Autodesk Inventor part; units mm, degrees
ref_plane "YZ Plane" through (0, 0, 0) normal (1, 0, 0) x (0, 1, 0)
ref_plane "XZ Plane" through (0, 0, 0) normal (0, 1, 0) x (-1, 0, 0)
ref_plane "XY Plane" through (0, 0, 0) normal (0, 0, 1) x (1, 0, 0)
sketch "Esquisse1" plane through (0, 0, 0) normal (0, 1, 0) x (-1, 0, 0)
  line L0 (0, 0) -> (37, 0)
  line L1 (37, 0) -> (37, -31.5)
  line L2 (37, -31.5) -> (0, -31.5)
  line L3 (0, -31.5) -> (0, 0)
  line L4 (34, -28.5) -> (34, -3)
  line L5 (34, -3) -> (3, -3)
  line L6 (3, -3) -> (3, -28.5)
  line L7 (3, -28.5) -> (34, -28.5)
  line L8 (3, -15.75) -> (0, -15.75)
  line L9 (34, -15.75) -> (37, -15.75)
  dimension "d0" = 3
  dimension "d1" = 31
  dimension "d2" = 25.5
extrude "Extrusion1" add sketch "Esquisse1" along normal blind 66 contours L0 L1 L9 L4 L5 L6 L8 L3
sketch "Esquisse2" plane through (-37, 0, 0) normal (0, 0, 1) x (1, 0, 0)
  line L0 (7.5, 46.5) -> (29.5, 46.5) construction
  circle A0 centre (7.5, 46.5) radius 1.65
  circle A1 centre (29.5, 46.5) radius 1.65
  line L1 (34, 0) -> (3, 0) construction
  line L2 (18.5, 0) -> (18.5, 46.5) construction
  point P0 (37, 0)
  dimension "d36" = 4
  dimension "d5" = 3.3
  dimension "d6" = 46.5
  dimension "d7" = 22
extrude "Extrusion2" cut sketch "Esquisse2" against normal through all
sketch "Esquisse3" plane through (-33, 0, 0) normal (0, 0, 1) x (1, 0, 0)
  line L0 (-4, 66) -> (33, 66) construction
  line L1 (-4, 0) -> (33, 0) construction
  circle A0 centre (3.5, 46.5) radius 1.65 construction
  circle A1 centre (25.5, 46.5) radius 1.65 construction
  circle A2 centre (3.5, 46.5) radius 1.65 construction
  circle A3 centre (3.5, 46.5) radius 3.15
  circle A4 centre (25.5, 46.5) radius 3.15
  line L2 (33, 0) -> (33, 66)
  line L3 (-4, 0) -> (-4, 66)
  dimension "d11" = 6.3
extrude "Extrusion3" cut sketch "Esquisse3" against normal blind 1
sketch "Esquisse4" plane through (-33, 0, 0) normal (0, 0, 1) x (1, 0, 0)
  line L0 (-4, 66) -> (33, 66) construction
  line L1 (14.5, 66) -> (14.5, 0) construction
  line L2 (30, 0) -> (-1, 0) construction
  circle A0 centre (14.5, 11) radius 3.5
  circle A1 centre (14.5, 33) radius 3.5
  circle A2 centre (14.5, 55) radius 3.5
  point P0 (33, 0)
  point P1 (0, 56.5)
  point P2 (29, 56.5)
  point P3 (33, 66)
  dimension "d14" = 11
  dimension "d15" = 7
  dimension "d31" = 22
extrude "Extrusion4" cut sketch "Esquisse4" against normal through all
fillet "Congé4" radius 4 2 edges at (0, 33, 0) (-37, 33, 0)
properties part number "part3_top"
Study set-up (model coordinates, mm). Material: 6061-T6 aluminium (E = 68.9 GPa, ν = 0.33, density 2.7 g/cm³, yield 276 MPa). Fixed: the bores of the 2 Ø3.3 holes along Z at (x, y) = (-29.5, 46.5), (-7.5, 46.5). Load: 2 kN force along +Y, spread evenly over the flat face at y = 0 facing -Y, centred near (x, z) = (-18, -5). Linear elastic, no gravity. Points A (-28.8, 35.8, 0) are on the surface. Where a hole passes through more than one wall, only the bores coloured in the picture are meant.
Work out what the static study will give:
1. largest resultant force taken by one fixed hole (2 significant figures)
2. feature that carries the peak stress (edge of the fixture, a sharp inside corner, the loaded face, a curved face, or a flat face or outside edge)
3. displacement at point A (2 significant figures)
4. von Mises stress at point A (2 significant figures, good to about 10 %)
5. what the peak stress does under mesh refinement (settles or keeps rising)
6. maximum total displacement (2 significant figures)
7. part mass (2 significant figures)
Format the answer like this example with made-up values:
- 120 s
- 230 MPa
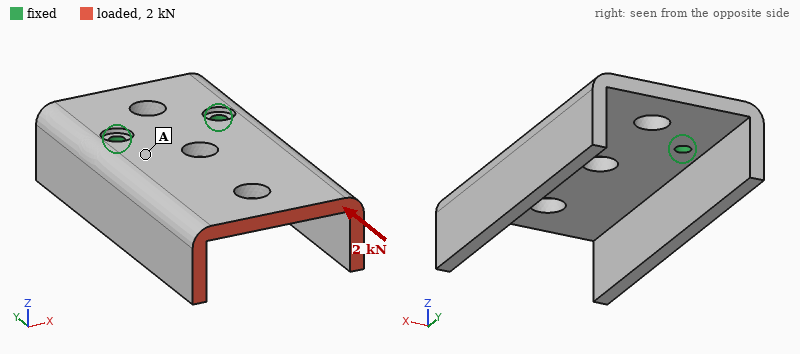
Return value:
- 1.0 kN
- edge of the fixture
- 0.045 mm
- 19 MPa
- keeps rising
- 0.25 mm
- 31 g
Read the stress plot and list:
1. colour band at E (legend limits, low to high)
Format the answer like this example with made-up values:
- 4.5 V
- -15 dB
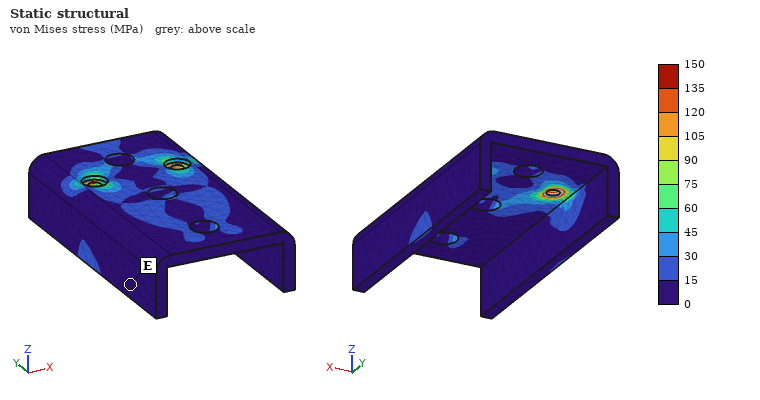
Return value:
- 0 to 15 MPa
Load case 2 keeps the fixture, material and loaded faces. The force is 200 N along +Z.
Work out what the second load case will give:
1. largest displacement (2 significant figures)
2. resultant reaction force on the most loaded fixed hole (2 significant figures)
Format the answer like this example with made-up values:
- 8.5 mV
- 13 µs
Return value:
- 0.41 mm
- 100 N
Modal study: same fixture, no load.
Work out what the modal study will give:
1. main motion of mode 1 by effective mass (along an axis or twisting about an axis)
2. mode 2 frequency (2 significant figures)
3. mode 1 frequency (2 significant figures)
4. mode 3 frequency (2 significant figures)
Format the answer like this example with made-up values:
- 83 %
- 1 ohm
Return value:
- along Z
- 2200 Hz
- 1300 Hz
- 4900 Hz
